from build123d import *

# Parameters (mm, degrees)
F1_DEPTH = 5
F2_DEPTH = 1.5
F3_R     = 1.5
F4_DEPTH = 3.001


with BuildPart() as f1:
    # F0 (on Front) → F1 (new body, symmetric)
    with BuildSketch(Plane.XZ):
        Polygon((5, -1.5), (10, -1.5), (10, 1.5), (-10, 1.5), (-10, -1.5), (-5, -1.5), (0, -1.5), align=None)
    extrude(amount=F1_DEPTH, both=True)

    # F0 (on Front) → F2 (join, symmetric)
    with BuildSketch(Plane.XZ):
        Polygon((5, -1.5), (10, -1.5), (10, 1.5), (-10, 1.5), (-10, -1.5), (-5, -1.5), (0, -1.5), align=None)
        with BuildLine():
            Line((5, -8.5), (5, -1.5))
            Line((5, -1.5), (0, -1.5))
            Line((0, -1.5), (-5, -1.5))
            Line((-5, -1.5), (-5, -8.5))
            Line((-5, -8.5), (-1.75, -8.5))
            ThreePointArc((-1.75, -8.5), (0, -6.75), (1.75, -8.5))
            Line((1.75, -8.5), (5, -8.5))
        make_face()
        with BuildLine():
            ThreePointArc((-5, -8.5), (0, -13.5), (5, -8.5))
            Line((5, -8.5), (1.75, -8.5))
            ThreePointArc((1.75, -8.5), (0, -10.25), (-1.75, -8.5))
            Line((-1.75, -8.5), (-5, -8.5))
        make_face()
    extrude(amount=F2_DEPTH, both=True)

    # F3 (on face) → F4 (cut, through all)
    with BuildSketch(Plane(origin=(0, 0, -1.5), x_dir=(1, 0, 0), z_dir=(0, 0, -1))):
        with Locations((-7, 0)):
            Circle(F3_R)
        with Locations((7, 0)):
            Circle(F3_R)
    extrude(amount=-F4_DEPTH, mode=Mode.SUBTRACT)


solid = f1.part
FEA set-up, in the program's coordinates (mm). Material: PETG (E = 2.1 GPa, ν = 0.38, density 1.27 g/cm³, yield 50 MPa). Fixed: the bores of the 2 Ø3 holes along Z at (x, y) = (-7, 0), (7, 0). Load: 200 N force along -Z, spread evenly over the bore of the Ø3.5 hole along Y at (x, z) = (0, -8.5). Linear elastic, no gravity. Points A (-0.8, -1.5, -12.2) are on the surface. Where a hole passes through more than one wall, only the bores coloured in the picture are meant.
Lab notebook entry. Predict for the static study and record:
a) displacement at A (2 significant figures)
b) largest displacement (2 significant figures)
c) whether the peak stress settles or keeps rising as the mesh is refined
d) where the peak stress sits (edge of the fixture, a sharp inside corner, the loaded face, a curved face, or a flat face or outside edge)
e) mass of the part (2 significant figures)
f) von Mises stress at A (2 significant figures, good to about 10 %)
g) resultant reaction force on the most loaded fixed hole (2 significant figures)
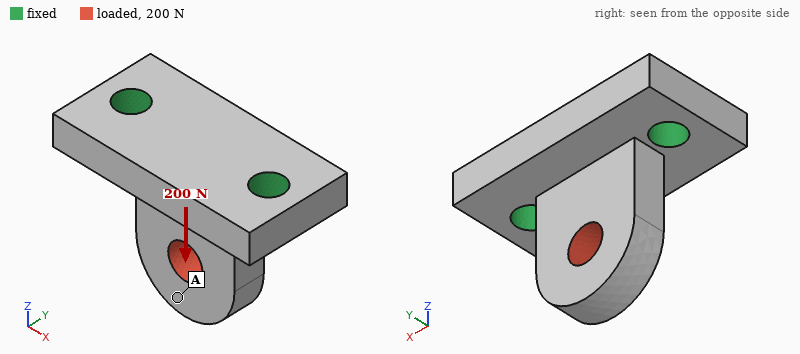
61 µm
66 µm
keeps rising
edge of the fixture
1.1 g
4.8 MPa
100 N
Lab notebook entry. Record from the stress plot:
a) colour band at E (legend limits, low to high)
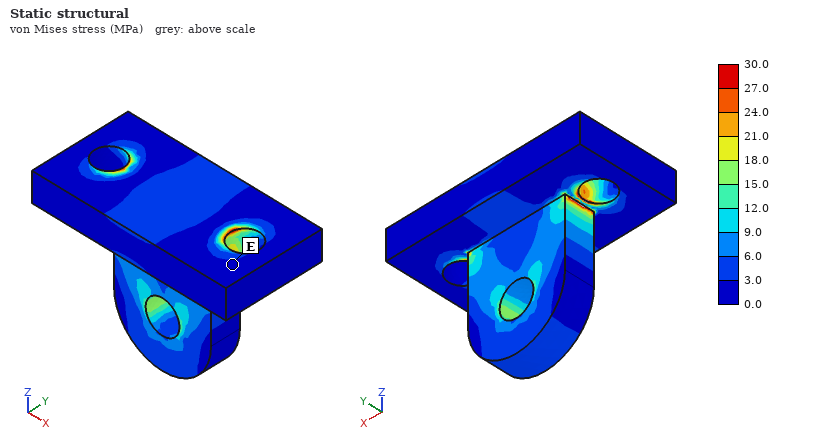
0.0 to 3.0 MPa
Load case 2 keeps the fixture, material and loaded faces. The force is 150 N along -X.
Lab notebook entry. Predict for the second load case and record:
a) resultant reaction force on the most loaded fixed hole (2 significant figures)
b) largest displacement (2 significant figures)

140 N
0.20 mm
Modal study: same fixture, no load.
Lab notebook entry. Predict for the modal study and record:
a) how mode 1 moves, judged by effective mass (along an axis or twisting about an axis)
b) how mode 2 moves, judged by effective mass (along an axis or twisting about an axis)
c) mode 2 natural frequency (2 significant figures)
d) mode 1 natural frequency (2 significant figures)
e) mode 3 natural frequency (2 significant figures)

along Y
along X
9400 Hz
3800 Hz
10 kHz
